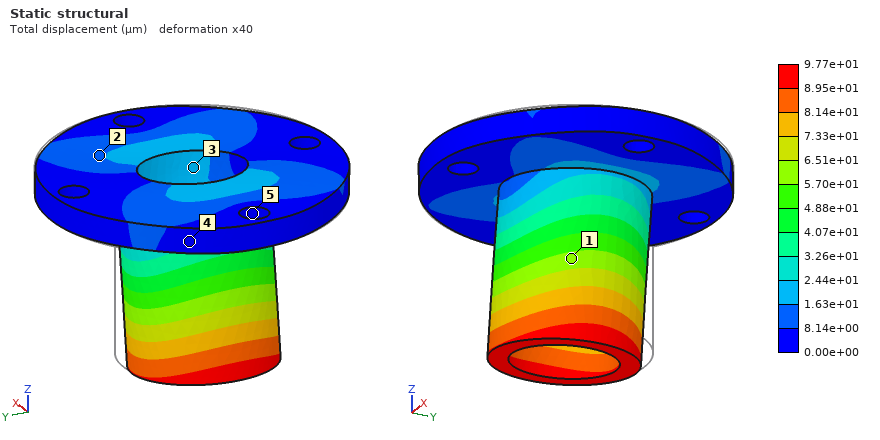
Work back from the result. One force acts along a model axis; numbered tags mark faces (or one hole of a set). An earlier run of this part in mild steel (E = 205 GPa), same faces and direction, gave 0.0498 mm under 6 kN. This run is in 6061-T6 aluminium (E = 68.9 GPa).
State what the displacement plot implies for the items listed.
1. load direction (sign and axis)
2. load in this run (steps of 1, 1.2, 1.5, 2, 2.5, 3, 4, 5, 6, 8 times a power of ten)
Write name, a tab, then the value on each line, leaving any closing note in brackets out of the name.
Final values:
load direction	-X
load in this run	4 kN
